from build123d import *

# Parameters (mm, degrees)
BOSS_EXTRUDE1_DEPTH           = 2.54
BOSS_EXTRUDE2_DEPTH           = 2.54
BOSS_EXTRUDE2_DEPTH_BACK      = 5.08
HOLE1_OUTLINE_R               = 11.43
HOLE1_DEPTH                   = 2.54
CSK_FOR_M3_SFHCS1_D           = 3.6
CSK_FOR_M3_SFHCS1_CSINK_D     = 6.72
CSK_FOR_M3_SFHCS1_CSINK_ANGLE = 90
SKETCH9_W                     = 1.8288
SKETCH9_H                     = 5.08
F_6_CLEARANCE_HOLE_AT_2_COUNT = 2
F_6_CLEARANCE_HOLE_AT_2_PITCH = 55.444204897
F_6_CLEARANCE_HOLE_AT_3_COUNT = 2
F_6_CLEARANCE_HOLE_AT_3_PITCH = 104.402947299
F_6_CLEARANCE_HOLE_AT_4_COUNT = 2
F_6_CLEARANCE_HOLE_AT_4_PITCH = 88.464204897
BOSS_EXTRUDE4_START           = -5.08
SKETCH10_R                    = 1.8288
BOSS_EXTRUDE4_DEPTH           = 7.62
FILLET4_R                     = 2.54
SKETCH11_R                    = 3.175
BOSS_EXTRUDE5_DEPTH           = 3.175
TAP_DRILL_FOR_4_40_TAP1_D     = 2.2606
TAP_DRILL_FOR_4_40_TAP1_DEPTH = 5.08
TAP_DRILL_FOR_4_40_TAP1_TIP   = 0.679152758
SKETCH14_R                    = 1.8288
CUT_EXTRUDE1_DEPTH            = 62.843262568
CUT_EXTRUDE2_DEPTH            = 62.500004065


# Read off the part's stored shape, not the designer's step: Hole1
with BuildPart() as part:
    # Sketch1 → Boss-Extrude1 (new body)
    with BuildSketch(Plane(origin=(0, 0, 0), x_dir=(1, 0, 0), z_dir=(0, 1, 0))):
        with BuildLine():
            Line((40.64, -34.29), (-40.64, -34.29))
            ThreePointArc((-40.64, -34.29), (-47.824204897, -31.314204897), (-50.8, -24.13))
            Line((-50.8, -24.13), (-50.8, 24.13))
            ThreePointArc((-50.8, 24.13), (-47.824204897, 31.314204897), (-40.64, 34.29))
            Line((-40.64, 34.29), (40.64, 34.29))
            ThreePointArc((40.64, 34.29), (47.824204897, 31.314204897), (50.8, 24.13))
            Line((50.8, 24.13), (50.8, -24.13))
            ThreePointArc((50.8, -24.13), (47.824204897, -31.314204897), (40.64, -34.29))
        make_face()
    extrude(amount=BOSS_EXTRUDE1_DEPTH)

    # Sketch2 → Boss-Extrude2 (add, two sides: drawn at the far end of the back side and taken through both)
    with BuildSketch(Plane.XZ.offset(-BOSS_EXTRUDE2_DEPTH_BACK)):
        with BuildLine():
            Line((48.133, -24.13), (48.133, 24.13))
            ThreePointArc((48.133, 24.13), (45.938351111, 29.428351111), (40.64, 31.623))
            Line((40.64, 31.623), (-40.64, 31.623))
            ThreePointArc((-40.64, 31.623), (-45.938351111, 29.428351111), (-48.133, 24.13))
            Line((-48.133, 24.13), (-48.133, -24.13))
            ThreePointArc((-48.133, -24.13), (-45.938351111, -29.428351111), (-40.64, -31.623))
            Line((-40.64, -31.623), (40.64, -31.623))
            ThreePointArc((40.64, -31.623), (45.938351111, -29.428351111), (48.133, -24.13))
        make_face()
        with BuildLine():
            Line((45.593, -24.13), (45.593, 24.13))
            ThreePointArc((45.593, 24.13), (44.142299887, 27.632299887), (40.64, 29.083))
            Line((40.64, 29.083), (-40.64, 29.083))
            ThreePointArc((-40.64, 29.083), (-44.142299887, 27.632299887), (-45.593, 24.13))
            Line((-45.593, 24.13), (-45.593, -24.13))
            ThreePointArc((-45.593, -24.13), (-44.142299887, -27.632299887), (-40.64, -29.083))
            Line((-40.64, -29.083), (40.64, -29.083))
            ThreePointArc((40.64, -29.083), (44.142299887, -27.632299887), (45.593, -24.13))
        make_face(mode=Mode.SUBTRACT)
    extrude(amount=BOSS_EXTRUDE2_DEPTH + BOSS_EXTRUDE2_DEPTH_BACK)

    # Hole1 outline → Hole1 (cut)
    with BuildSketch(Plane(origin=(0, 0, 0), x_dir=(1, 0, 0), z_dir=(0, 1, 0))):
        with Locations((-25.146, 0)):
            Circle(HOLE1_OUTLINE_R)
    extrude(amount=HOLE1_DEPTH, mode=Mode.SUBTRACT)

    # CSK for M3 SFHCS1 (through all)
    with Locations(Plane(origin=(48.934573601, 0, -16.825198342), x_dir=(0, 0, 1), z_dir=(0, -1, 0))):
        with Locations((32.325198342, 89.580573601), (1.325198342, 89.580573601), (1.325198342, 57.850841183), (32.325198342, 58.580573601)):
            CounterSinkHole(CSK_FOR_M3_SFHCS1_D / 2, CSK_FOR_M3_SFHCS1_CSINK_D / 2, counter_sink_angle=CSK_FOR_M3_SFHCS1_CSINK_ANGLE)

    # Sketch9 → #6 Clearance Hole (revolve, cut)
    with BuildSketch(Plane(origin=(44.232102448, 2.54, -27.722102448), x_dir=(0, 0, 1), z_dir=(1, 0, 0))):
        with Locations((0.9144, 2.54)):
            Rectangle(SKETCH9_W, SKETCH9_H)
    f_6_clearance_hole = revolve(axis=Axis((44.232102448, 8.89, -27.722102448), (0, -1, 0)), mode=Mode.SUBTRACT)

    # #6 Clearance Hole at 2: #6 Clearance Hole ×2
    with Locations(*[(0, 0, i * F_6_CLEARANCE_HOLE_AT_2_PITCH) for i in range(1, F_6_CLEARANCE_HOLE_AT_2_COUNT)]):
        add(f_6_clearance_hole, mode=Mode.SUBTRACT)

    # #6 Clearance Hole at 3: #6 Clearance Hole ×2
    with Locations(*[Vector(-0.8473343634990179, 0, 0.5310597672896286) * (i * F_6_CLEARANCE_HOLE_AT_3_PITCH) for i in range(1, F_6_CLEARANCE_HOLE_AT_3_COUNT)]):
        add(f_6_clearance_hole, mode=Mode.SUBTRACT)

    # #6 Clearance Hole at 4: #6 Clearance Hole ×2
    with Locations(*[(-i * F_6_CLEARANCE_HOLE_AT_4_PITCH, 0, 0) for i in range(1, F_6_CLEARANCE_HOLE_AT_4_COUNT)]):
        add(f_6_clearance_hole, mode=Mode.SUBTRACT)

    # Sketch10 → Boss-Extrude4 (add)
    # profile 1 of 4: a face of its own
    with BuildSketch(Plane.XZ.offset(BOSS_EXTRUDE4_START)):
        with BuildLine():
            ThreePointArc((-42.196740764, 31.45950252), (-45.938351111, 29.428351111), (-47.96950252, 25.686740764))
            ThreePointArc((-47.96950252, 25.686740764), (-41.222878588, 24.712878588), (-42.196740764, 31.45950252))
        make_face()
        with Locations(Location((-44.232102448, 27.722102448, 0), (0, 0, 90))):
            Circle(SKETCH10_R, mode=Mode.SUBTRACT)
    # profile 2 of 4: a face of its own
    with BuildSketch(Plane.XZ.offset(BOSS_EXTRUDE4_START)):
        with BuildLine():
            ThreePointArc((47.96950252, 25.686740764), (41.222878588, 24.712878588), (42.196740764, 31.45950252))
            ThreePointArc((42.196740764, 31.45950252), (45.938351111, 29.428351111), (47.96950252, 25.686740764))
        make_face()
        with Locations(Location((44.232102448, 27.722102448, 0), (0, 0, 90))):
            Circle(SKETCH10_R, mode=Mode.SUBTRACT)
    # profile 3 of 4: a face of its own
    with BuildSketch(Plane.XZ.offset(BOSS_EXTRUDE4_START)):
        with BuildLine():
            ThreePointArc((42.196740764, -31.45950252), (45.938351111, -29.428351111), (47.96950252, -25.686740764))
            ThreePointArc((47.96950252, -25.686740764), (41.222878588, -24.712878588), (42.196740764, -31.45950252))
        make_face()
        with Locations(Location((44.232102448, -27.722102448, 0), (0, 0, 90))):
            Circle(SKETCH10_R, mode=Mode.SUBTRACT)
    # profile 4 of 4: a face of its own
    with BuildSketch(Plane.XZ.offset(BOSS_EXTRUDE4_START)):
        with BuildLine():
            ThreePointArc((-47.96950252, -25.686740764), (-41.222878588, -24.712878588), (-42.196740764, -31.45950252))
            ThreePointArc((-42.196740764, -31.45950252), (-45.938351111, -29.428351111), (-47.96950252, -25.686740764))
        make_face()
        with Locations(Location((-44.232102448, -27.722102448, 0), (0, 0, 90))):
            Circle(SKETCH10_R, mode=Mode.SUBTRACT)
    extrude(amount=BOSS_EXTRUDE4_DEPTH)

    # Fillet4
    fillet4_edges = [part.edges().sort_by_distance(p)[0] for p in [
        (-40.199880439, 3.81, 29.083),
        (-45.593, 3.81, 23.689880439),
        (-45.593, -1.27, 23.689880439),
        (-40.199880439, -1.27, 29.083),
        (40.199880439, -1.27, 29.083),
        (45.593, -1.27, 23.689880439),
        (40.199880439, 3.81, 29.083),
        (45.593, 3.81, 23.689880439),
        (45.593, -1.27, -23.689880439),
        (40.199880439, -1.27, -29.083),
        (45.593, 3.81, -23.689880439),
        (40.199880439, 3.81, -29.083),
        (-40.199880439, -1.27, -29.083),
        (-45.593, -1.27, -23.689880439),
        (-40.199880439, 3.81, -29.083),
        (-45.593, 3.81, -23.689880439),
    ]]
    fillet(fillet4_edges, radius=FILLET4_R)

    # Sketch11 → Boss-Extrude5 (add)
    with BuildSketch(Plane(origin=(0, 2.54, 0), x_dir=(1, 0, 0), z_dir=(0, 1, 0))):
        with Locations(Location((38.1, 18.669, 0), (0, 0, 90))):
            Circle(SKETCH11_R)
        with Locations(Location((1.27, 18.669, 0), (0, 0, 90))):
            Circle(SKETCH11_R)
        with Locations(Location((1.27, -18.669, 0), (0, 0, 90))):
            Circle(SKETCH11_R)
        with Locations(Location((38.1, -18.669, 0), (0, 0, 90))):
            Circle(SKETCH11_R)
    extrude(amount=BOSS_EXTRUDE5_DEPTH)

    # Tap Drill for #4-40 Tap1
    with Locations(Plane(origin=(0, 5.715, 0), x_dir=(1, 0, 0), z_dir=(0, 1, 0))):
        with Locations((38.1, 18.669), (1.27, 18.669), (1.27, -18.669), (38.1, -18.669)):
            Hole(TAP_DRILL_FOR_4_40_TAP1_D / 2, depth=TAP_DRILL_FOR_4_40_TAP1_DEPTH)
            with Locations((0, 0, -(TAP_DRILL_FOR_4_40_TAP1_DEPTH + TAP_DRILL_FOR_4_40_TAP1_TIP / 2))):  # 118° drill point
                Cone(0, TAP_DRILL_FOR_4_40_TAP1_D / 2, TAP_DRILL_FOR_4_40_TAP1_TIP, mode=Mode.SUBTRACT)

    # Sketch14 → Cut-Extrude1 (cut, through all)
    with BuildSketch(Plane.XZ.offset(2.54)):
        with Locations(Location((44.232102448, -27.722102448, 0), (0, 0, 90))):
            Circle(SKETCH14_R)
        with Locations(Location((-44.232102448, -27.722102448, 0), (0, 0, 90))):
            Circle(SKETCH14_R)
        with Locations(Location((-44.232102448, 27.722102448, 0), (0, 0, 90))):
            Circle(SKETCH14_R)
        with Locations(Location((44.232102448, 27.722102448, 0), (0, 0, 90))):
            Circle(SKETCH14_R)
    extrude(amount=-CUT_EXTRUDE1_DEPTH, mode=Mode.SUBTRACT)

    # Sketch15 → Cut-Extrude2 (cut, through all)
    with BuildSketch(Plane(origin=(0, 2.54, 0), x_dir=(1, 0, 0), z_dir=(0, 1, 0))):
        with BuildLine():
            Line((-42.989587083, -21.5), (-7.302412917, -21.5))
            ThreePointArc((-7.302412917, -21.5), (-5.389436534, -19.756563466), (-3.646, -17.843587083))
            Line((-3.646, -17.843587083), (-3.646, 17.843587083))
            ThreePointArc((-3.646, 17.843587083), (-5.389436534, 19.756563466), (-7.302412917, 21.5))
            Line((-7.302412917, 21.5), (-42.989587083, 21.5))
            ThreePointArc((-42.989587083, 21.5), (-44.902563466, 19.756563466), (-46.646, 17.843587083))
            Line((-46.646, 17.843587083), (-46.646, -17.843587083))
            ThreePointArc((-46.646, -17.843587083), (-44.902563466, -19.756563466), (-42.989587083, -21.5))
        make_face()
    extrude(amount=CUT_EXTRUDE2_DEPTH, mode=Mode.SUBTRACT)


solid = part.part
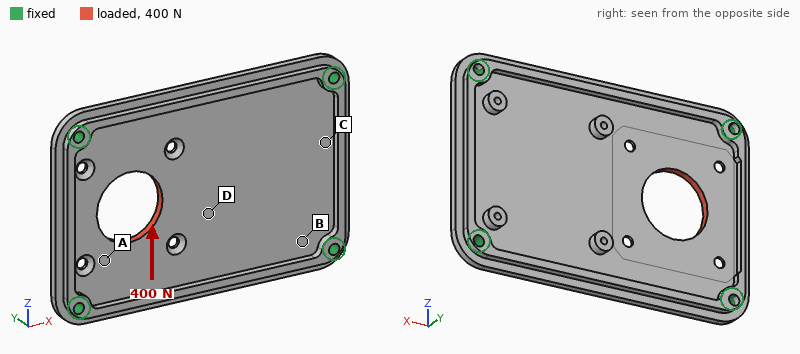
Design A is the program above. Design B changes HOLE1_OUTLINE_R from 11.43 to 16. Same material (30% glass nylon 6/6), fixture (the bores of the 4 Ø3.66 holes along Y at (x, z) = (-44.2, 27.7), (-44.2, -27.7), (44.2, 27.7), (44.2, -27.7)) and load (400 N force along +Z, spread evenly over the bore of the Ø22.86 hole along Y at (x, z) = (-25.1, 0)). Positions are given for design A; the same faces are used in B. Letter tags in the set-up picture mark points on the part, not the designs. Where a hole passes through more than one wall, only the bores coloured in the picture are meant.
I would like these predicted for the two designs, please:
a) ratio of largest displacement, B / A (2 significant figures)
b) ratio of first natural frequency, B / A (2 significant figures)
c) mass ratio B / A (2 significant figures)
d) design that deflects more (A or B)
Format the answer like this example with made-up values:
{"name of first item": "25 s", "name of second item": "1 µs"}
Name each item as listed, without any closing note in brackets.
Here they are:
{"ratio of largest displacement, B / A": "1.1", "ratio of first natural frequency, B / A": "1.00", "mass ratio B / A": "0.95", "design that deflects more": "B"}
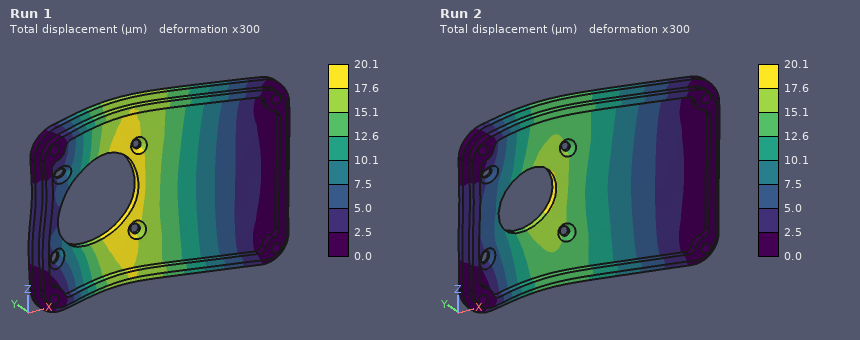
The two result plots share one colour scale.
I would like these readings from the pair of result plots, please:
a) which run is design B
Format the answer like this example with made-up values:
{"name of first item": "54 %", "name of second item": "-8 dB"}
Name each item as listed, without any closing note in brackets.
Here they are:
{"which run is design B": "Run 1"}
